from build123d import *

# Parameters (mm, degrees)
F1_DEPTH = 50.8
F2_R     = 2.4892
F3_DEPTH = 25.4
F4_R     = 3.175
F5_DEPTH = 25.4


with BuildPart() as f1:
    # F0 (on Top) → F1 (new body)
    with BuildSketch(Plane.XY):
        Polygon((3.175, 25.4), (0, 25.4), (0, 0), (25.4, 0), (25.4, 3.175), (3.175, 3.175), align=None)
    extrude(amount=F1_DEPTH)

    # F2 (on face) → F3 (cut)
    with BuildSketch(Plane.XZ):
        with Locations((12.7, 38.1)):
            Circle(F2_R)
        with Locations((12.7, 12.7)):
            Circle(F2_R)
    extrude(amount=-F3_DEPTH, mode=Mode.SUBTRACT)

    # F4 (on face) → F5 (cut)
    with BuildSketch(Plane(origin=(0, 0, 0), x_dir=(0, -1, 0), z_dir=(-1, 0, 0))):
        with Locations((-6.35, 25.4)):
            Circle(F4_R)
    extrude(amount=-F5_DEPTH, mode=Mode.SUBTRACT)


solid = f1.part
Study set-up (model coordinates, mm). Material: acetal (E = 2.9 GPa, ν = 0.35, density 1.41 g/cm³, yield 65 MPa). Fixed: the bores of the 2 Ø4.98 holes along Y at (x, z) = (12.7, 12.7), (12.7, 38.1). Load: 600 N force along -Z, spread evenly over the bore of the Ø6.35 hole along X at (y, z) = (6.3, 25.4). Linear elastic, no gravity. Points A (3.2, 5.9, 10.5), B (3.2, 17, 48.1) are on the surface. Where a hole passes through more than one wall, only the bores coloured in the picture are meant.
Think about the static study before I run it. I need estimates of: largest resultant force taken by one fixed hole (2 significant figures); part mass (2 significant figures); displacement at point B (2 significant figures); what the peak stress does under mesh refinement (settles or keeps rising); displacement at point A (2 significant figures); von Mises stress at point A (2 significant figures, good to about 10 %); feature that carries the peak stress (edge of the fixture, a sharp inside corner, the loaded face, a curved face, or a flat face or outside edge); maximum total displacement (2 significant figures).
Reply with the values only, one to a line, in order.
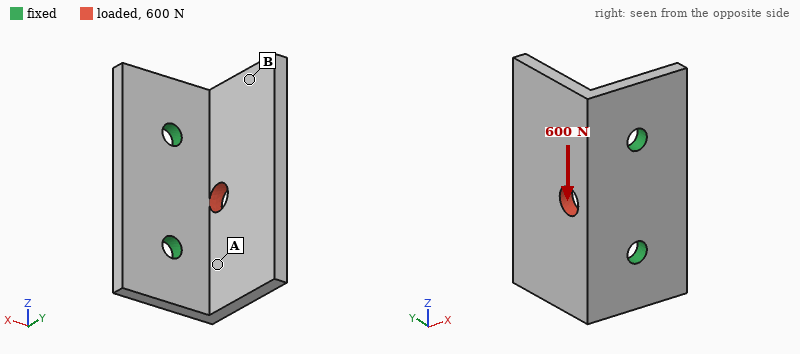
380 N
11 g
0.35 mm
keeps rising
0.17 mm
8.9 MPa
edge of the fixture
0.47 mm
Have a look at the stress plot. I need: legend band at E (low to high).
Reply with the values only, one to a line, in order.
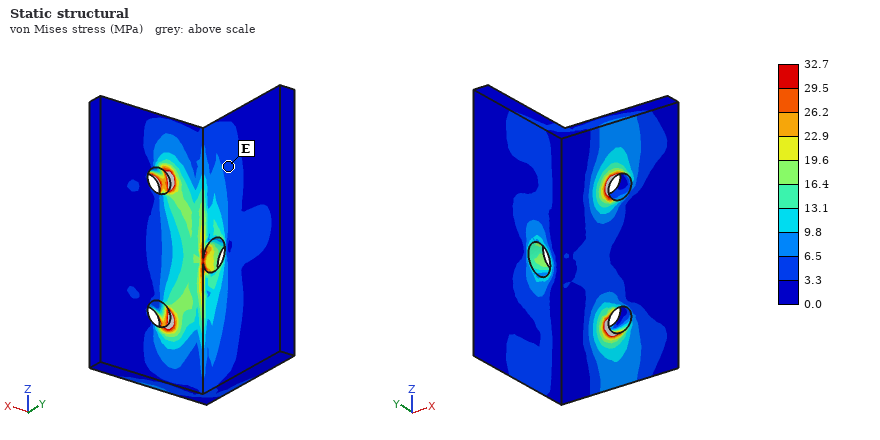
3.3 to 6.5 MPa
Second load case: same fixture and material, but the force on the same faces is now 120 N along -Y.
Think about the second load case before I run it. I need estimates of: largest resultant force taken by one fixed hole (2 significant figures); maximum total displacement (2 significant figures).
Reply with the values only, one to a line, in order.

60 N
0.45 mm
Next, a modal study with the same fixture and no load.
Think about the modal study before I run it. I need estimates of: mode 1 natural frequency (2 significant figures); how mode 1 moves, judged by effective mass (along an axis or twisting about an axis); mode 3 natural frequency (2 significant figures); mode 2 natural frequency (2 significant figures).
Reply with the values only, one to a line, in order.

770 Hz
along X
2100 Hz
1300 Hz
